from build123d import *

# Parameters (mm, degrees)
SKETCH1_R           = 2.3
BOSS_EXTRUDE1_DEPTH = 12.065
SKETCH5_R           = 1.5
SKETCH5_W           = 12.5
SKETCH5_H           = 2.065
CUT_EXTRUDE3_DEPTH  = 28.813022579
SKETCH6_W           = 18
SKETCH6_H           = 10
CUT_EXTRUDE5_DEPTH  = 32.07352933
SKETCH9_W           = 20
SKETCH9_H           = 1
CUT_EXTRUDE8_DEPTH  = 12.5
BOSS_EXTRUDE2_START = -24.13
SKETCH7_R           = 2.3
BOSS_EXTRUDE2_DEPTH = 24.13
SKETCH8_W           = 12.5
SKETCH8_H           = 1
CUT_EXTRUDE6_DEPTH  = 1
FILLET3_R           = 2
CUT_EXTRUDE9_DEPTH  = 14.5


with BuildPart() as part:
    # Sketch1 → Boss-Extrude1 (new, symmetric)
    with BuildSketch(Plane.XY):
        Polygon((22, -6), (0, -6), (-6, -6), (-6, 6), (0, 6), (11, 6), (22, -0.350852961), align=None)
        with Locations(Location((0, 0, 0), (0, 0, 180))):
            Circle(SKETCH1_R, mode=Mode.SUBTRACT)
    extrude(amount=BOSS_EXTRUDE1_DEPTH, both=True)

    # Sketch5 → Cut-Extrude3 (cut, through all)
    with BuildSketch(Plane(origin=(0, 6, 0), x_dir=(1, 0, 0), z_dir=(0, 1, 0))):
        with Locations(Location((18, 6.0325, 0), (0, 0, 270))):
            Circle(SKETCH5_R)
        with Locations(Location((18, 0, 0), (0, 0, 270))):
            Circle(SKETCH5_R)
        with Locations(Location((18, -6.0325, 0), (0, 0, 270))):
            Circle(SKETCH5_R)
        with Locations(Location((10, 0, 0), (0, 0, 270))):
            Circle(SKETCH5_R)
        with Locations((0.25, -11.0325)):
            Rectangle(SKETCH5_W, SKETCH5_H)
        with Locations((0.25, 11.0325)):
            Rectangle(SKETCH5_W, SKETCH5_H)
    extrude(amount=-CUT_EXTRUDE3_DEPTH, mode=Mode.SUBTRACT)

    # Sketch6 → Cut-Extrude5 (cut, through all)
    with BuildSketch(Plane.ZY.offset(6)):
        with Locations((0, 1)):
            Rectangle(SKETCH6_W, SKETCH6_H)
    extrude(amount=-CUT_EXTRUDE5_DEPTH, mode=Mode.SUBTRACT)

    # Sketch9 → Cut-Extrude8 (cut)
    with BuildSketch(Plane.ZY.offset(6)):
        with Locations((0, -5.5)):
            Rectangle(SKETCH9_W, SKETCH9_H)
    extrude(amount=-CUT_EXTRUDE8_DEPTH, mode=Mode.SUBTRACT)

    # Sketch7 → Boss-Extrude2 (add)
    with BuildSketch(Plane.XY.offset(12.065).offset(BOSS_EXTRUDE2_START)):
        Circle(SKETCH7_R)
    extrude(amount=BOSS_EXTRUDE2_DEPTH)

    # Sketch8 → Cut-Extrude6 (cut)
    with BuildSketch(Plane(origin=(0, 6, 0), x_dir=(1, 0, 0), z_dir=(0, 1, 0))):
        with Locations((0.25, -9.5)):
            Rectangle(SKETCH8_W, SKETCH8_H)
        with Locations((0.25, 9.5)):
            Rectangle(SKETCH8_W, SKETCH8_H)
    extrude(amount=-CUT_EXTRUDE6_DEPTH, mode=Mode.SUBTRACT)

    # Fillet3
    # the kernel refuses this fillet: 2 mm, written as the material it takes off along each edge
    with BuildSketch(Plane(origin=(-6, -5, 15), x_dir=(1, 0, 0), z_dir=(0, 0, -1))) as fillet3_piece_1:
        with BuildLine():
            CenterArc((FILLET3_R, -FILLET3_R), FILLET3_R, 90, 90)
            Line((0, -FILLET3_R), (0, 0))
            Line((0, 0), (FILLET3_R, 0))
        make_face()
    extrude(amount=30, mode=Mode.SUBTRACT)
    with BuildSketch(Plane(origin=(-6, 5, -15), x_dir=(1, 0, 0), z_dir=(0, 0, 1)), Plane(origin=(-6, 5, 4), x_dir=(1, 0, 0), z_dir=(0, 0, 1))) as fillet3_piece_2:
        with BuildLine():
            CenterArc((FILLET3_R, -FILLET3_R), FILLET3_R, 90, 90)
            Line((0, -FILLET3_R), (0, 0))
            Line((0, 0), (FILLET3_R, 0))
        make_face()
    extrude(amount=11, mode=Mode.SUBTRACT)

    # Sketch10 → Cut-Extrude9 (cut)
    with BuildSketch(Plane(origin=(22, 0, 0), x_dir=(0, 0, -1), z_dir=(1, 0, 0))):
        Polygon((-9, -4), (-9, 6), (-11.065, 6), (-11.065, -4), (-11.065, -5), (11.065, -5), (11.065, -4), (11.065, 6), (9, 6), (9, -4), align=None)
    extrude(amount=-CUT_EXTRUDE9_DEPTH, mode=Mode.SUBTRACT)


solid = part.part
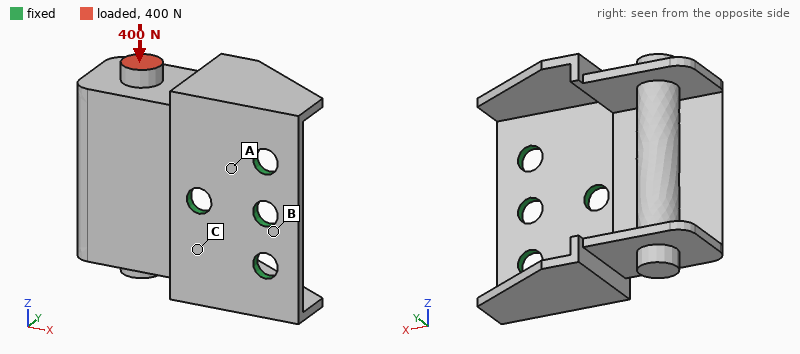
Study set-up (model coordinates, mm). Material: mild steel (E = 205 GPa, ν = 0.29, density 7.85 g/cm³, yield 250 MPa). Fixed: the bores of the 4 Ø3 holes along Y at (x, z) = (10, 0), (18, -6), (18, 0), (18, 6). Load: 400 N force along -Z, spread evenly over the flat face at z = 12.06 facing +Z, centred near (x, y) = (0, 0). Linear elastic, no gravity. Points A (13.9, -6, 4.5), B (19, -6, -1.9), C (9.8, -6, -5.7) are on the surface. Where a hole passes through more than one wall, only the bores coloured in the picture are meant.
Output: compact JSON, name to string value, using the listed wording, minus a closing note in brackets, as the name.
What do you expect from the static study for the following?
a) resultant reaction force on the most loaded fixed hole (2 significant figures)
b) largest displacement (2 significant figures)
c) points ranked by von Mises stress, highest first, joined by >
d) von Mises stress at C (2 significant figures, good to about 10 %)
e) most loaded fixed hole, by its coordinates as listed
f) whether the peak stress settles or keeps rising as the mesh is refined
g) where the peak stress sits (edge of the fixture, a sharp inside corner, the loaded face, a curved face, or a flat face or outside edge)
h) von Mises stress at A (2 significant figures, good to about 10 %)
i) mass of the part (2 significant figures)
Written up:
{"resultant reaction force on the most loaded fixed hole": "490 N", "largest displacement": "81 µm", "points ranked by von Mises stress, highest first, joined by >": "A > C > B", "von Mises stress at C": "45 MPa", "most loaded fixed hole, by its coordinates as listed": "(10, 0)", "whether the peak stress settles or keeps rising as the mesh is refined": "keeps rising", "where the peak stress sits": "edge of the fixture", "von Mises stress at A": "79 MPa", "mass of the part": "12 g"}
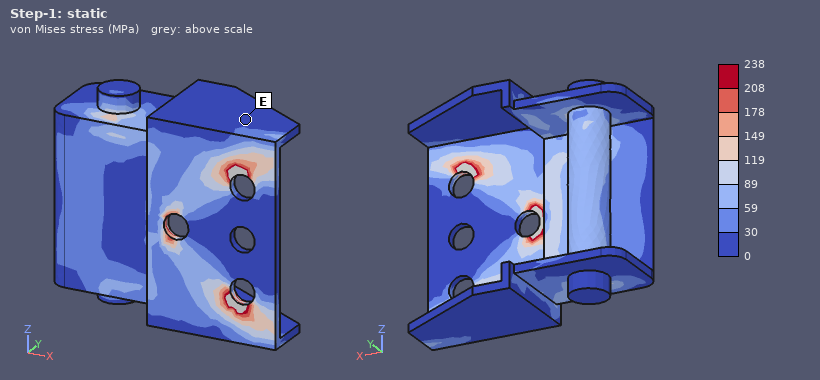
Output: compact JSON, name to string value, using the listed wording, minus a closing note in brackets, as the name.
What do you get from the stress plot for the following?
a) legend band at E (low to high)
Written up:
{"legend band at E": "0 to 30 MPa"}
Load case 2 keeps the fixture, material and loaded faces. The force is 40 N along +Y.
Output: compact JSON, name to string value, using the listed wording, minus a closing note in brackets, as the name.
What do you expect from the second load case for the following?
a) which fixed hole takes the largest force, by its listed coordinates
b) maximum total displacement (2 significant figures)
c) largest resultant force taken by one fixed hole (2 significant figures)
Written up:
{"which fixed hole takes the largest force, by its listed coordinates": "(10, 0)", "maximum total displacement": "37 µm", "largest resultant force taken by one fixed hole": "71 N"}
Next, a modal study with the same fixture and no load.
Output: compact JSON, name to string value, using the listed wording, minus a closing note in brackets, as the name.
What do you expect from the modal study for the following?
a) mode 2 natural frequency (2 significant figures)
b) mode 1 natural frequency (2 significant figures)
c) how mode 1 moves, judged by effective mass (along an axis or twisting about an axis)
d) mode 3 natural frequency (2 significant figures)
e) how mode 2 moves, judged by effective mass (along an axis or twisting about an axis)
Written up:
{"mode 2 natural frequency": "3600 Hz", "mode 1 natural frequency": "3200 Hz", "how mode 1 moves, judged by effective mass": "along Y", "mode 3 natural frequency": "7900 Hz", "how mode 2 moves, judged by effective mass": "along Z"}
